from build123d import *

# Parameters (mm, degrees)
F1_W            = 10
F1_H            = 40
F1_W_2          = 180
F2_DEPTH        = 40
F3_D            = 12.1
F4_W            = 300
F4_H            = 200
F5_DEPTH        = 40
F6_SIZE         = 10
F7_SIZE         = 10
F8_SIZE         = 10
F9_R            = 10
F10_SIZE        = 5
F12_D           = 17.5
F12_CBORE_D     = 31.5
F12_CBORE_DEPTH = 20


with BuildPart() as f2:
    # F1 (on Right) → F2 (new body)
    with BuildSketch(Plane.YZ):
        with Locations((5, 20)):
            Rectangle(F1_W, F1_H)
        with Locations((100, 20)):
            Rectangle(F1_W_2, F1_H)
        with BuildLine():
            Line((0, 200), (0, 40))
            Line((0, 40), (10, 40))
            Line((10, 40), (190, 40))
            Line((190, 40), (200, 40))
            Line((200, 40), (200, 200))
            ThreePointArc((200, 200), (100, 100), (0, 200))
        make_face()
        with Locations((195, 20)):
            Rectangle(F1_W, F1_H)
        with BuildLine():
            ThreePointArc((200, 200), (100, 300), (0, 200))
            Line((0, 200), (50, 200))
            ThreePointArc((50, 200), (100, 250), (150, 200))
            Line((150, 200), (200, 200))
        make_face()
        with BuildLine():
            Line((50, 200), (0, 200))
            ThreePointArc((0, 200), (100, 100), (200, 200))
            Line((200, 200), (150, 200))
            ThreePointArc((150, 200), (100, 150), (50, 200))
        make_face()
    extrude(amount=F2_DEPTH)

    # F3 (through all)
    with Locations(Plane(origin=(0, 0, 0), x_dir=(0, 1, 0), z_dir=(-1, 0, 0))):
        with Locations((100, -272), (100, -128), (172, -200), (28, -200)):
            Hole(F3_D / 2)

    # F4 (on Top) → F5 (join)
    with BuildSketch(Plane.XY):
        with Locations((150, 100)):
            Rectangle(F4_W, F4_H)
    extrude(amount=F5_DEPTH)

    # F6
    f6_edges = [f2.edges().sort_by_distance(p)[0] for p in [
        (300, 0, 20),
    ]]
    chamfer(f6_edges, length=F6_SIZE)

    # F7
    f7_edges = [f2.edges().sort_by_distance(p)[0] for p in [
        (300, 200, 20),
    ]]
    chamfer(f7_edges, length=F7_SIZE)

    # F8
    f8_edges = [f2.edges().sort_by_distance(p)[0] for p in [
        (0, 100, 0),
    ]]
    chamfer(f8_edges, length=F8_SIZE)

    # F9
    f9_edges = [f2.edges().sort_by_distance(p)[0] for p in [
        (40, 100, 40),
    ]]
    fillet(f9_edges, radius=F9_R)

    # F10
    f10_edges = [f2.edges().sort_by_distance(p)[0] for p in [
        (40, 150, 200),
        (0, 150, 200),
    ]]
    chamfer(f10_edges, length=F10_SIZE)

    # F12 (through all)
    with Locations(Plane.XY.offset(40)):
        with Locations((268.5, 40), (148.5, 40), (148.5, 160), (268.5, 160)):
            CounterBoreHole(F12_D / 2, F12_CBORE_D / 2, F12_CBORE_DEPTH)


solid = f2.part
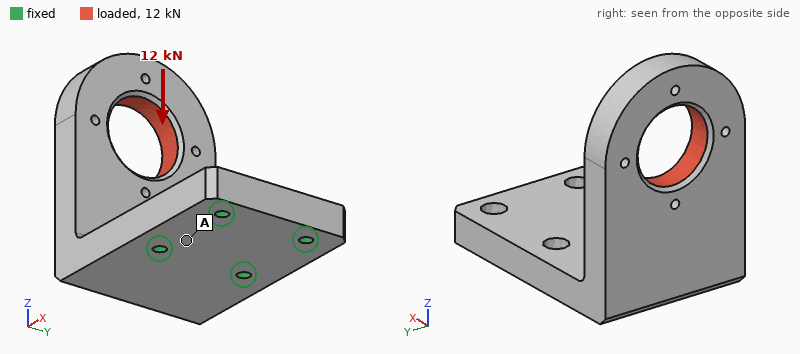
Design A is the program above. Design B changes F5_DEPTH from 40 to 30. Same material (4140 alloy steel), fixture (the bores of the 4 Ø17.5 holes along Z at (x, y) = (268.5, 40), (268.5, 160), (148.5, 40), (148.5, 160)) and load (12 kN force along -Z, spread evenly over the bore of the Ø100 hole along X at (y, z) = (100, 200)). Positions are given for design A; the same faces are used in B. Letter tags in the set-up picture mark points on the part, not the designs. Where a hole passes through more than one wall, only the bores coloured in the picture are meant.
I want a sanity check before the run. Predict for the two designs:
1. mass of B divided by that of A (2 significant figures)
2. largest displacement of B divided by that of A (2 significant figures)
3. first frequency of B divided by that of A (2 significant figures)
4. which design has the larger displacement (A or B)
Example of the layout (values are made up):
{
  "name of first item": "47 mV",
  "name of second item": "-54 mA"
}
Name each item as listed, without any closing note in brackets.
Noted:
{
  "mass of B divided by that of A": "0.87",
  "largest displacement of B divided by that of A": "2.1",
  "first frequency of B divided by that of A": "0.71",
  "which design has the larger displacement": "B"
}
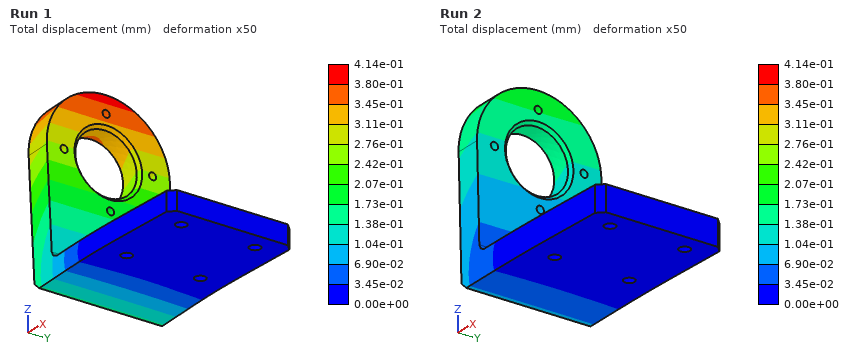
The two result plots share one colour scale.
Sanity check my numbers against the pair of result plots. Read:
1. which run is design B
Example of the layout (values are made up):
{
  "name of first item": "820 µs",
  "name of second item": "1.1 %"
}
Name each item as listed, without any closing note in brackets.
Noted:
{
  "which run is design B": "Run 1"
}
